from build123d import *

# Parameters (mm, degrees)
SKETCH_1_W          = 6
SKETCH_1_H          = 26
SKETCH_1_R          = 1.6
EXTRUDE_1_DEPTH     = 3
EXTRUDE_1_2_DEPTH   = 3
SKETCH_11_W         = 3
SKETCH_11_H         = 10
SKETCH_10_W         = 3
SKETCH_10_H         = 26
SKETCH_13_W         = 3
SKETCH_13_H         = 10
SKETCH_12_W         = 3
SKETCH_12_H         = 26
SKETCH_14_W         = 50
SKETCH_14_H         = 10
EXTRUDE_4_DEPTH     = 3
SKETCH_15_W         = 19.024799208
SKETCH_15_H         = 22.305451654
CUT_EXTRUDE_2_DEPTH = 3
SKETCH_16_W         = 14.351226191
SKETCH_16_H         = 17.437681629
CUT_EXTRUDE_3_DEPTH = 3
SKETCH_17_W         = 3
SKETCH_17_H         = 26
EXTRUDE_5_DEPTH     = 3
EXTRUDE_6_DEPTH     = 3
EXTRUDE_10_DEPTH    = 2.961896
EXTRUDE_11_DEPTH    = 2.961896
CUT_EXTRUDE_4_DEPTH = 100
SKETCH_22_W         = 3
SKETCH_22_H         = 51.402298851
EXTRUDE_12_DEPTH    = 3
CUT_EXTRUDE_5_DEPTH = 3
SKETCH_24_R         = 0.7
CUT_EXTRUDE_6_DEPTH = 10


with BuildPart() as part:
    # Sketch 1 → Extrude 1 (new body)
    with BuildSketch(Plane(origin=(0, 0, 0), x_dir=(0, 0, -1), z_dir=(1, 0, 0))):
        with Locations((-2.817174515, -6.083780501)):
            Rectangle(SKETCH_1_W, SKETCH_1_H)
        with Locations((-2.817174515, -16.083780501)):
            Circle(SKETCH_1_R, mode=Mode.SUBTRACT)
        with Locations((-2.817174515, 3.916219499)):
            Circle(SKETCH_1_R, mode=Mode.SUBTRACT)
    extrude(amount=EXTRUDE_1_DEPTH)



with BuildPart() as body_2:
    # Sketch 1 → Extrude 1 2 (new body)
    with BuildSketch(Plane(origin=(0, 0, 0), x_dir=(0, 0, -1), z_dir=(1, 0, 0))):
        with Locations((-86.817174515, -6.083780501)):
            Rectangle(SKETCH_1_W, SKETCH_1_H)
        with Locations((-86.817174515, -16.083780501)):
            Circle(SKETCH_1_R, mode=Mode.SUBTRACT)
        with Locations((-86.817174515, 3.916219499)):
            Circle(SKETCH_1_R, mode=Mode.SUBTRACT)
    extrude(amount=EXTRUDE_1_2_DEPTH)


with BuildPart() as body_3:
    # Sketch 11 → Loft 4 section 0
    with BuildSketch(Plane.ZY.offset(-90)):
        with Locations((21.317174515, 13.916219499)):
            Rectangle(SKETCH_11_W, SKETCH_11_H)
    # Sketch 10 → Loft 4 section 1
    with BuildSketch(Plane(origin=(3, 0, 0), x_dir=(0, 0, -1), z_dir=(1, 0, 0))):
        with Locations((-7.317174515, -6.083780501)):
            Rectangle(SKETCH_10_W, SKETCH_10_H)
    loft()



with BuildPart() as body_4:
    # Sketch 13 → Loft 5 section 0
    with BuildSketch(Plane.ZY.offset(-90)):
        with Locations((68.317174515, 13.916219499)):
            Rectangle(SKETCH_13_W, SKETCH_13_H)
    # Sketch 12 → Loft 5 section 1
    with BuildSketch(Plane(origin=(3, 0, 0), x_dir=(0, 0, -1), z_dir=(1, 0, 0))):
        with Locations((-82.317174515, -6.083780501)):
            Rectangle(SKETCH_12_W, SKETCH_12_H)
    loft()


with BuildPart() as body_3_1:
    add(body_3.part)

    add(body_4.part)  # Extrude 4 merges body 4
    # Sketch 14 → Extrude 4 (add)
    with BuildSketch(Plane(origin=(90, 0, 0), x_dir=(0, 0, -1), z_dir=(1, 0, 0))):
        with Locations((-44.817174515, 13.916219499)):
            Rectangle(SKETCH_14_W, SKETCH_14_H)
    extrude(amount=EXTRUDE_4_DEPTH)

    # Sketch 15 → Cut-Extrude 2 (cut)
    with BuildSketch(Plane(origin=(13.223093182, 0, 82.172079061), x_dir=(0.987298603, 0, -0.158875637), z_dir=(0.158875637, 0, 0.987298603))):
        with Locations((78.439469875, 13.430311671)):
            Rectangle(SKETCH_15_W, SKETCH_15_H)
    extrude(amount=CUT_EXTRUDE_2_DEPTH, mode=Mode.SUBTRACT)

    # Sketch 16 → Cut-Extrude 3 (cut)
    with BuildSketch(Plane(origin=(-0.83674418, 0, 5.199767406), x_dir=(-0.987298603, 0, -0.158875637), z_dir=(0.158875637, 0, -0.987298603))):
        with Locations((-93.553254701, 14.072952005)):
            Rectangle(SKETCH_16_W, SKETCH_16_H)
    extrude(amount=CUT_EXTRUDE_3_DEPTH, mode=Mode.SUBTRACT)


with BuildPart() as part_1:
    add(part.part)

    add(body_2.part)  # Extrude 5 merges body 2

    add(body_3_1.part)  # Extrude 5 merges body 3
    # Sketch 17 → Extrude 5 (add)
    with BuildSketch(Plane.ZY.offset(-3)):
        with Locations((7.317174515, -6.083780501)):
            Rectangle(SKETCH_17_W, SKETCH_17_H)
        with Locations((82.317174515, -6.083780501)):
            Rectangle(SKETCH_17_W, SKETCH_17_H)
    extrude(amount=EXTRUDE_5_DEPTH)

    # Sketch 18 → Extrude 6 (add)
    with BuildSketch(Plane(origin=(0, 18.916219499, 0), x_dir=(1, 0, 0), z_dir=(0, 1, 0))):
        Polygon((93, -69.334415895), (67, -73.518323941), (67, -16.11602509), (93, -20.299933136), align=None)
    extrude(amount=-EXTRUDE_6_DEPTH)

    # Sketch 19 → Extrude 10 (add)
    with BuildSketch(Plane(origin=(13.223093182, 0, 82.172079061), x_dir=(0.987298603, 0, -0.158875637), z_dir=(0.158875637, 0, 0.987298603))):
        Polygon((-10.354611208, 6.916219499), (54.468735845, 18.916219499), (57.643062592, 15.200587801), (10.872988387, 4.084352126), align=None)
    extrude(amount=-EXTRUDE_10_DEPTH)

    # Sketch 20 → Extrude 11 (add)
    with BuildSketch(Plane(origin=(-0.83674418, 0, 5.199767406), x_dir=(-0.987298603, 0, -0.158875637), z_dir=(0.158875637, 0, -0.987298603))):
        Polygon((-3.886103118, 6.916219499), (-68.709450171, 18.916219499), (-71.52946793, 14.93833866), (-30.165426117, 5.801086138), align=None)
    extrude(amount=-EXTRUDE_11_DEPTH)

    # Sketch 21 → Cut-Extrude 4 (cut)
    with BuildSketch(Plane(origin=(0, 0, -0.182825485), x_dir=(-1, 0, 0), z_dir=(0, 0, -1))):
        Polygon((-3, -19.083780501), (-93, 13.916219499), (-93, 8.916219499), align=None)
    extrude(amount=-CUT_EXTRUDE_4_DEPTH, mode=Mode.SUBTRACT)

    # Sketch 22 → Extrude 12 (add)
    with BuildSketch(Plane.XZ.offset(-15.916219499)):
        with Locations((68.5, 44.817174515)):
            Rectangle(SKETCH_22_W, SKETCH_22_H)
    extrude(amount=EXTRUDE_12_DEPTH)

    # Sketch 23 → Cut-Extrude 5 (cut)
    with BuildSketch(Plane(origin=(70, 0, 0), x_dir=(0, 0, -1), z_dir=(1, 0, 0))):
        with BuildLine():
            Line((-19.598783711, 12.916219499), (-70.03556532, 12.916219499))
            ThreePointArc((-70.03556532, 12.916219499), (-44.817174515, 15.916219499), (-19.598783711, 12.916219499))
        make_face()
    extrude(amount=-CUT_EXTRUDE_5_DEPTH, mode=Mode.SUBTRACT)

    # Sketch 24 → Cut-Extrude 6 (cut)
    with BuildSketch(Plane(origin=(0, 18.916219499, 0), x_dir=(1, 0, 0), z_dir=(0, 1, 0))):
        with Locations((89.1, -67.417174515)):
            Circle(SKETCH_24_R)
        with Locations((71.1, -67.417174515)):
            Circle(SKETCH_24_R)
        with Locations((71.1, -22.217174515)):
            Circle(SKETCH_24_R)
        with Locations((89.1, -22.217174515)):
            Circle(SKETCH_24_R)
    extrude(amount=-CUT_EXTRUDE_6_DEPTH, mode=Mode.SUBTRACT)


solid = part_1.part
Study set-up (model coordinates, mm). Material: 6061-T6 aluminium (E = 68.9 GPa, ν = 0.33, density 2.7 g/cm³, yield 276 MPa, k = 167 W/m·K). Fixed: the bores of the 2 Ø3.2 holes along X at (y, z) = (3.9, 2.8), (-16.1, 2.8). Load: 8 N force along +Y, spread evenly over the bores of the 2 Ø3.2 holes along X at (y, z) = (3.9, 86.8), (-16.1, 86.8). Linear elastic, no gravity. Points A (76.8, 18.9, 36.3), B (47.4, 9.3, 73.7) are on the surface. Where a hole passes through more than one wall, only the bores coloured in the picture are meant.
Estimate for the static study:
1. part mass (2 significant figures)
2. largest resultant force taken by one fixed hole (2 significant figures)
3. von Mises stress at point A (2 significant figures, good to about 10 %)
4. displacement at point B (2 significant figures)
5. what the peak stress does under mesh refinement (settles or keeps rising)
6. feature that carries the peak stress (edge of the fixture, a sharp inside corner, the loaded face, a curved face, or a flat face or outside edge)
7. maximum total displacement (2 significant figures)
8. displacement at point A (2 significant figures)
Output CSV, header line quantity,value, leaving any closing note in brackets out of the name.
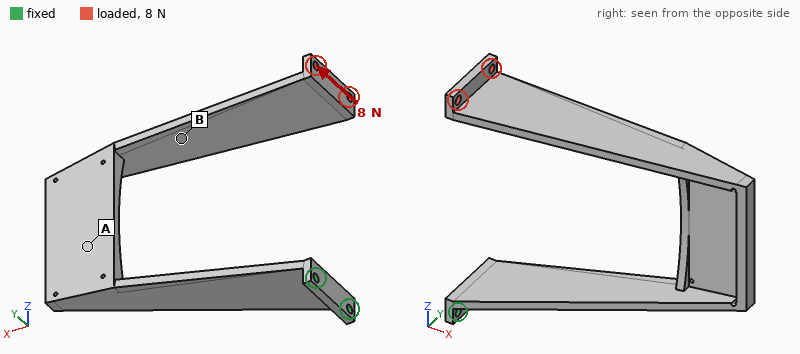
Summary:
quantity,value
part mass,40 g
largest resultant force taken by one fixed hole,34 N
von Mises stress at point A,12 MPa
displacement at point B,0.89 mm
what the peak stress does under mesh refinement,keeps rising
feature that carries the peak stress,a sharp inside corner
maximum total displacement,1.5 mm
displacement at point A,0.29 mm
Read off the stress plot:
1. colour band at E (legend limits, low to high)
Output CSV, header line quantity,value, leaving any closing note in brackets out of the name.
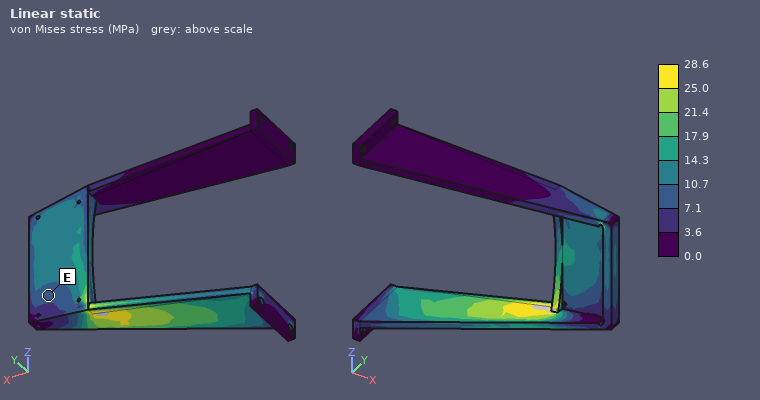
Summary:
quantity,value
colour band at E,7.1 to 10.7 MPa
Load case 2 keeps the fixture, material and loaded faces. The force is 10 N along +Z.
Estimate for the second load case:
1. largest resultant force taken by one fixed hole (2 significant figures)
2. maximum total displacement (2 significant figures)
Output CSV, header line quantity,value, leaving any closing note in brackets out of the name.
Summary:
quantity,value
largest resultant force taken by one fixed hole,5.1 N
maximum total displacement,1.6 mm
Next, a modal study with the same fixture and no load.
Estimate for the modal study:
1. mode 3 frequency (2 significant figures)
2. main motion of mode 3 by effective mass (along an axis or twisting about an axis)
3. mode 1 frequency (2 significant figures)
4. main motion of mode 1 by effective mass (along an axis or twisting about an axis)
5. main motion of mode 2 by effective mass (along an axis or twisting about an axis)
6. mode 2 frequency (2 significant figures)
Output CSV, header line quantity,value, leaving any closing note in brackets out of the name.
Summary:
quantity,value
mode 3 frequency,220 Hz
main motion of mode 3 by effective mass,along Z
mode 1 frequency,91 Hz
main motion of mode 1 by effective mass,along X
main motion of mode 2 by effective mass,along Y
mode 2 frequency,120 Hz
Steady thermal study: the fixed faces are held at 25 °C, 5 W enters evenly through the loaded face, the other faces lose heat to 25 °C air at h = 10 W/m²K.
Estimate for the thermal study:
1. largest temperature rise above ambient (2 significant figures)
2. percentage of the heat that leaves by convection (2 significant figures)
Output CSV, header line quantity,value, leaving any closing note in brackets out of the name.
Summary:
quantity,value
largest temperature rise above ambient,63 K
percentage of the heat that leaves by convection,60 %
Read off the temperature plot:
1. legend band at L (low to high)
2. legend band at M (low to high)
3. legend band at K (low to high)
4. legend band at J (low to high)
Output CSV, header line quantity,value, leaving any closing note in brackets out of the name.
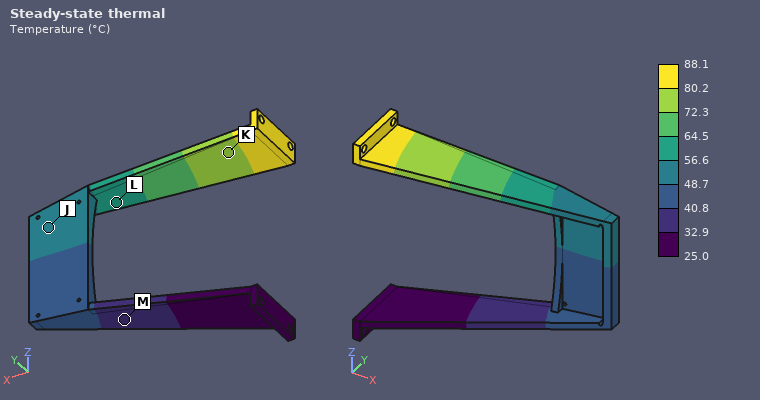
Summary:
quantity,value
legend band at L,56.6 to 64.5 °C
legend band at M,32.9 to 40.8 °C
legend band at K,72.3 to 80.2 °C
legend band at J,48.7 to 56.6 °C
